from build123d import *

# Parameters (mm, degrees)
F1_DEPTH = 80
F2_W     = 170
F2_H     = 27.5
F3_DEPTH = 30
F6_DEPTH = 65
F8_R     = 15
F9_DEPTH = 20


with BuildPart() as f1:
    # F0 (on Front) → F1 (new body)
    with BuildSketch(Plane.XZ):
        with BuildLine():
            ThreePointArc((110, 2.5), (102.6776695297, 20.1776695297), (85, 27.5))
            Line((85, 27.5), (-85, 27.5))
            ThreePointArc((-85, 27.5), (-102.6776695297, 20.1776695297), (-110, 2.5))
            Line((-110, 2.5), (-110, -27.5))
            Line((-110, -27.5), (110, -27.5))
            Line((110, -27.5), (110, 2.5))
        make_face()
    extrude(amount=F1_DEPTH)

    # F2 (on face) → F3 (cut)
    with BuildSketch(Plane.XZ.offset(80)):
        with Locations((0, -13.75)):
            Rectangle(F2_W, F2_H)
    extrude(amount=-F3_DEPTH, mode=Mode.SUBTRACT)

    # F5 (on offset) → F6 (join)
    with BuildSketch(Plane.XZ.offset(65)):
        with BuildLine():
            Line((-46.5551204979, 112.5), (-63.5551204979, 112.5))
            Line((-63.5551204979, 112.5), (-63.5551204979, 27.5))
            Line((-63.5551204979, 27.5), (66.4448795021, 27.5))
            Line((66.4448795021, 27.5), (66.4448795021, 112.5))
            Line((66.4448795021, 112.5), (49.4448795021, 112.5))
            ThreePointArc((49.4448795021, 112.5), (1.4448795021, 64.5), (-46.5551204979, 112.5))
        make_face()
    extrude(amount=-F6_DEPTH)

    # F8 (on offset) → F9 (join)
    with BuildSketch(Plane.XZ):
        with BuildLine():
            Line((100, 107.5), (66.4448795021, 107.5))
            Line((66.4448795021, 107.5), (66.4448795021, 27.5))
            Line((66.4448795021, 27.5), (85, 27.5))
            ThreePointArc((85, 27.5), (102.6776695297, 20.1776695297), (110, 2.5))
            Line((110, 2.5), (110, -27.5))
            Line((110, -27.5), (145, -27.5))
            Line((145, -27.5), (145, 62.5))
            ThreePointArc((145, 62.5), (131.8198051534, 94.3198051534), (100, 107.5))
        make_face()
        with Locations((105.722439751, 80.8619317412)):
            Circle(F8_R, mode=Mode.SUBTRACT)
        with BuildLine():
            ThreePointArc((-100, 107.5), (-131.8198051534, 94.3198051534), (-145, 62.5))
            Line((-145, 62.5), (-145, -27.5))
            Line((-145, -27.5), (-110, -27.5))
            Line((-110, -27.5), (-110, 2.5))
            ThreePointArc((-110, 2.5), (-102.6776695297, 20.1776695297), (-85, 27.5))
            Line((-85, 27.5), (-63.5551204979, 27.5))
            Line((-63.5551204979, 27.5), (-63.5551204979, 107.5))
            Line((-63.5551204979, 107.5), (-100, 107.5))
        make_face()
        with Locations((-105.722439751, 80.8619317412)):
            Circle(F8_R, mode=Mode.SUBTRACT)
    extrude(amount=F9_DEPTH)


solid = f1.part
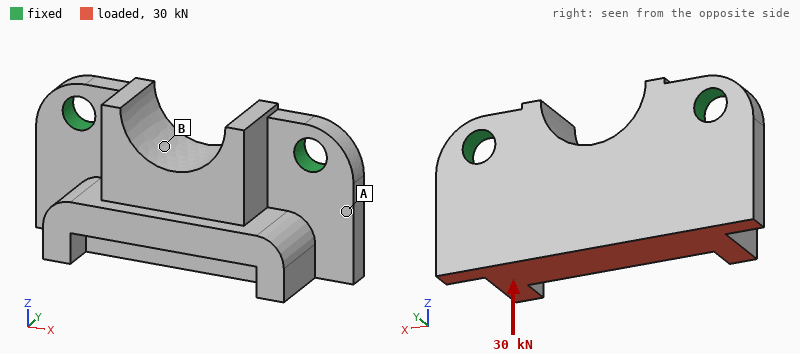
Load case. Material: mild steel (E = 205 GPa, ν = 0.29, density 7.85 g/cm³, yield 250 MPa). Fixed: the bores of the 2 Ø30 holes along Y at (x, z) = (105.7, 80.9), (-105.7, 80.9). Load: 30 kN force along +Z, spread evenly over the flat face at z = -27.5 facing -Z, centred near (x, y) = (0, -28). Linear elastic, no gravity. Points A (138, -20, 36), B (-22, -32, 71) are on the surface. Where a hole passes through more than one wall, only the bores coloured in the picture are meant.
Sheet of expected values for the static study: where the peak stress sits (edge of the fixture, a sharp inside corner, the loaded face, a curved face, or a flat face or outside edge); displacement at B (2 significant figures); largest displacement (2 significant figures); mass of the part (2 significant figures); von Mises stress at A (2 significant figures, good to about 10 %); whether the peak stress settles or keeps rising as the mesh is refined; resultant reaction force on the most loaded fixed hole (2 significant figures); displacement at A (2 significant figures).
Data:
edge of the fixture
13 µm
53 µm
12 kg
16 MPa
keeps rising
16 kN
8.6 µm
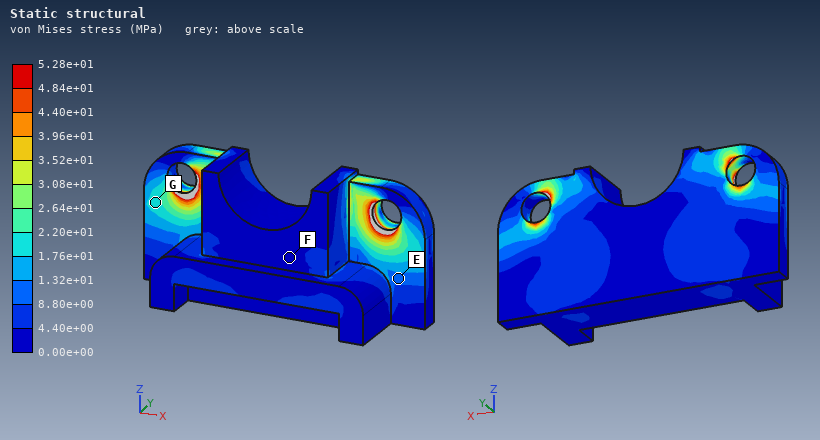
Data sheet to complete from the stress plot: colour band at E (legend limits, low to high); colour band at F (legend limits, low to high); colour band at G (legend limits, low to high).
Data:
8.80e+00 to 1.32e+01 MPa
0.00e+00 to 4.40e+00 MPa
1.76e+01 to 2.20e+01 MPa
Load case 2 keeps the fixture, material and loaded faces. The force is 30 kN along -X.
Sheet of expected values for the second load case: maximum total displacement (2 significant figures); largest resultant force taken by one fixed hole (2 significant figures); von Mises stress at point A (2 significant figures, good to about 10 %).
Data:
14 µm
21 kN
6.3 MPa
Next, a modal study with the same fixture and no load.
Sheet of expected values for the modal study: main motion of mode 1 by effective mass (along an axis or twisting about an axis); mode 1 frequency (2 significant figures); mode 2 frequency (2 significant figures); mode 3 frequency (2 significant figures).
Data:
along Y
840 Hz
2400 Hz
3000 Hz
